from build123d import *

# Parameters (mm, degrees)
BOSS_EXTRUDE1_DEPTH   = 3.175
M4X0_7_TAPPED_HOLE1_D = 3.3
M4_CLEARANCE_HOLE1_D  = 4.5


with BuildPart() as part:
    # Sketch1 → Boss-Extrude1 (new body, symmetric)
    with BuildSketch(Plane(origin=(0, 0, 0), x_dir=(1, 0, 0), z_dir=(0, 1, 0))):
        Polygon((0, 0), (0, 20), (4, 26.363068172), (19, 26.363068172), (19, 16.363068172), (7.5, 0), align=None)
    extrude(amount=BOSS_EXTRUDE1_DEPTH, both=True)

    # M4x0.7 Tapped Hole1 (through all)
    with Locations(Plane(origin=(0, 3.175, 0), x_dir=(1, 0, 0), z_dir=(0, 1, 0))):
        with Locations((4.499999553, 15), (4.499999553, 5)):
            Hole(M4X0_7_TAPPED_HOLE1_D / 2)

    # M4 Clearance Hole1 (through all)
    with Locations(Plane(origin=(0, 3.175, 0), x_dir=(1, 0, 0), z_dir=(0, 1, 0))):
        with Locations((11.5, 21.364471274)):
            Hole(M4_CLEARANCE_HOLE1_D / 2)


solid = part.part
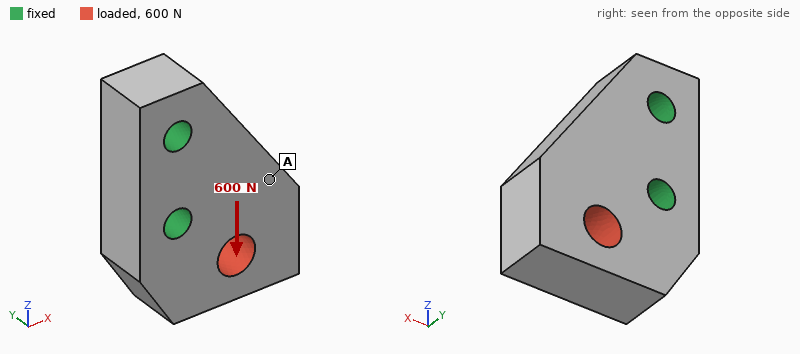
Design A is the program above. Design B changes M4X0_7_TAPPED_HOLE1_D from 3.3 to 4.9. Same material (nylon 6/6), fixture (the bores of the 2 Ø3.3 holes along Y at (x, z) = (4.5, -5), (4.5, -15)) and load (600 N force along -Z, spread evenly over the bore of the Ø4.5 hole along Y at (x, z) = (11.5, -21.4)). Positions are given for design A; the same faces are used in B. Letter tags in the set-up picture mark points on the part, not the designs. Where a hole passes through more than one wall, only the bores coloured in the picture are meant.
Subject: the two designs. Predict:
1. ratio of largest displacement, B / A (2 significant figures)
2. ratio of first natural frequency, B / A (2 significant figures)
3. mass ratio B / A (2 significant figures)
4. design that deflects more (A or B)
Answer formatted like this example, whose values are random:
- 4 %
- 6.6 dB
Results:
- 0.80
- 1.1
- 0.94
- A
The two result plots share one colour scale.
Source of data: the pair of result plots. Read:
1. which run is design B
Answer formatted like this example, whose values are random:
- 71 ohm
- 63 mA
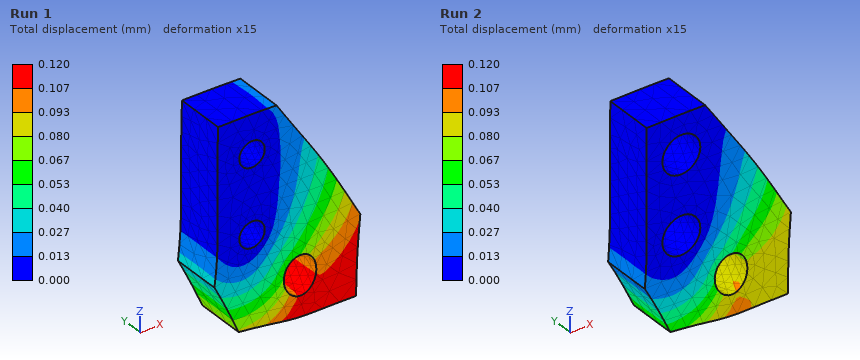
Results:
- Run 2
